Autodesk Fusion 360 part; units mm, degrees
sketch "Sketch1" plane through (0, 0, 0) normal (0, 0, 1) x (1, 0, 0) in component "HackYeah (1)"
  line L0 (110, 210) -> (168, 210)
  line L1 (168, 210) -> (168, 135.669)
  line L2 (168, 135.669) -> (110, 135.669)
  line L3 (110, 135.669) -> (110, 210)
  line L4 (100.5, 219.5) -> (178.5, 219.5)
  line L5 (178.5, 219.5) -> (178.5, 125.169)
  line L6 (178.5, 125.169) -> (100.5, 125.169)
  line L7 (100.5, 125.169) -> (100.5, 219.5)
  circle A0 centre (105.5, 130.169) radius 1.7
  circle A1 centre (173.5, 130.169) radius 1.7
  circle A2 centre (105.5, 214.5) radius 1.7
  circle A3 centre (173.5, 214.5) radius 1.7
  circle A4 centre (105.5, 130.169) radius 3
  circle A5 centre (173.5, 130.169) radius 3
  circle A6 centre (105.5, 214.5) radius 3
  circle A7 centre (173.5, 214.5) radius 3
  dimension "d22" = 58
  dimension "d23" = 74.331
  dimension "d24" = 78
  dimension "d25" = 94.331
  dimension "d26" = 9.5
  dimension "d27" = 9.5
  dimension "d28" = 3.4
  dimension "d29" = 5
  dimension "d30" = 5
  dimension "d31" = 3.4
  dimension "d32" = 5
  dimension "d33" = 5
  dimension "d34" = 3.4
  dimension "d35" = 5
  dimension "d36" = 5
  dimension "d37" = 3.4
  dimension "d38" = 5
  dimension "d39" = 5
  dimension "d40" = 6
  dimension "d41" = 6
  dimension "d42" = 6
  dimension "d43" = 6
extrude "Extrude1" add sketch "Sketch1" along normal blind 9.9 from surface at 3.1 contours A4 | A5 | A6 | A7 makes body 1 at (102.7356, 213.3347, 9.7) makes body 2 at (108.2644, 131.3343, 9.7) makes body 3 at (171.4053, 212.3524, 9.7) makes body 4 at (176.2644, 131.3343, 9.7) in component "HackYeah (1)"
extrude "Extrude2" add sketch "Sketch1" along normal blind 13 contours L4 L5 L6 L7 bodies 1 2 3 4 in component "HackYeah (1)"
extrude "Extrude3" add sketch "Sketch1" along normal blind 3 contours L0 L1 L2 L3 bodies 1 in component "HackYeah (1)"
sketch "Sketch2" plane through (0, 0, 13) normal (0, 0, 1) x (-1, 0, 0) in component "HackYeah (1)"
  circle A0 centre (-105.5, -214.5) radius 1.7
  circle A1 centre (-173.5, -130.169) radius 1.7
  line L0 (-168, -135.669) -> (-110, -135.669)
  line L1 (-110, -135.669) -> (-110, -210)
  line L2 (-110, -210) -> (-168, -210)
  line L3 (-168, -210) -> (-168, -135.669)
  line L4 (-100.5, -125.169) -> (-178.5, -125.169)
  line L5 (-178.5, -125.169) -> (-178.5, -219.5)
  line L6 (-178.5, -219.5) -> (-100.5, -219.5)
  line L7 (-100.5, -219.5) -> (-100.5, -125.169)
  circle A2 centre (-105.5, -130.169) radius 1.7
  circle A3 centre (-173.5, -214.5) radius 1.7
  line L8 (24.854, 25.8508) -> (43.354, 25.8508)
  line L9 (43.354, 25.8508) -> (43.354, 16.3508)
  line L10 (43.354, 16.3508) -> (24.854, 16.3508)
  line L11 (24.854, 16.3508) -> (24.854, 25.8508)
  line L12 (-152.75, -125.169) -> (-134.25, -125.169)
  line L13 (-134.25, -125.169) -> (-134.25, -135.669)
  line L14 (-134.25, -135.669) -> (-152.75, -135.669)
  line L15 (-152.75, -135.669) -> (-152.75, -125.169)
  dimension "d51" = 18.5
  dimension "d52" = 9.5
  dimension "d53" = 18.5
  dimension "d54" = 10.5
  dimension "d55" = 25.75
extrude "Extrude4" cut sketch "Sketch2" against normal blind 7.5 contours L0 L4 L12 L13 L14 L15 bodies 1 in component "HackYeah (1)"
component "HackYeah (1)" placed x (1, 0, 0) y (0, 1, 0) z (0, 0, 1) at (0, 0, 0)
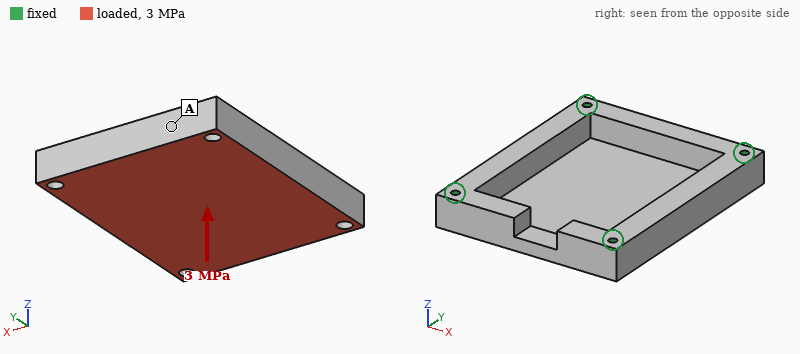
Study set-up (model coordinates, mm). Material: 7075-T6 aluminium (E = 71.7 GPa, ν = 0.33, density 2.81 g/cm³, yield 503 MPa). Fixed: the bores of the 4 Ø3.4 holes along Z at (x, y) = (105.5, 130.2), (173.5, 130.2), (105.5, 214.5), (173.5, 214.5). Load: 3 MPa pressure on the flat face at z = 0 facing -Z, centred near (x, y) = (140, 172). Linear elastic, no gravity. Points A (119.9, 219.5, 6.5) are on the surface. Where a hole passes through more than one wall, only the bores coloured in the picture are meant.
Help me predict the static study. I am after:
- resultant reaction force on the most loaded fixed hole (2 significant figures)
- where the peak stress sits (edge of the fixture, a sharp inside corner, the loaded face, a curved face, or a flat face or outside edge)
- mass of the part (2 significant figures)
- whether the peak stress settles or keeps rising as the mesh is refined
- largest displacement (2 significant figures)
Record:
8.2 kN
edge of the fixture
140 g
keeps rising
0.67 mm
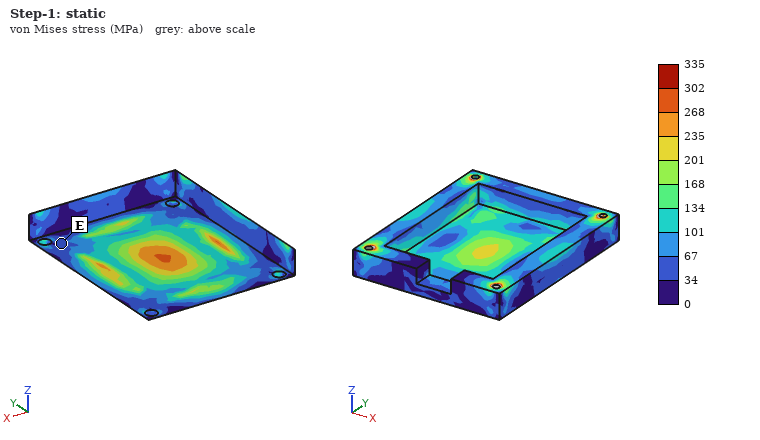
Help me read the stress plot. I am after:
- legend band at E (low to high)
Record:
34 to 67 MPa
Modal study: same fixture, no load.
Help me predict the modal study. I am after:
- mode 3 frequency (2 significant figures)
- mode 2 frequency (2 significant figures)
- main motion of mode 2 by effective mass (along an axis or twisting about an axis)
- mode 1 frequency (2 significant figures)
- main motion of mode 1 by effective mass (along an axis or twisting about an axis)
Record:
8100 Hz
6900 Hz
twisting about Y
4600 Hz
along Z
